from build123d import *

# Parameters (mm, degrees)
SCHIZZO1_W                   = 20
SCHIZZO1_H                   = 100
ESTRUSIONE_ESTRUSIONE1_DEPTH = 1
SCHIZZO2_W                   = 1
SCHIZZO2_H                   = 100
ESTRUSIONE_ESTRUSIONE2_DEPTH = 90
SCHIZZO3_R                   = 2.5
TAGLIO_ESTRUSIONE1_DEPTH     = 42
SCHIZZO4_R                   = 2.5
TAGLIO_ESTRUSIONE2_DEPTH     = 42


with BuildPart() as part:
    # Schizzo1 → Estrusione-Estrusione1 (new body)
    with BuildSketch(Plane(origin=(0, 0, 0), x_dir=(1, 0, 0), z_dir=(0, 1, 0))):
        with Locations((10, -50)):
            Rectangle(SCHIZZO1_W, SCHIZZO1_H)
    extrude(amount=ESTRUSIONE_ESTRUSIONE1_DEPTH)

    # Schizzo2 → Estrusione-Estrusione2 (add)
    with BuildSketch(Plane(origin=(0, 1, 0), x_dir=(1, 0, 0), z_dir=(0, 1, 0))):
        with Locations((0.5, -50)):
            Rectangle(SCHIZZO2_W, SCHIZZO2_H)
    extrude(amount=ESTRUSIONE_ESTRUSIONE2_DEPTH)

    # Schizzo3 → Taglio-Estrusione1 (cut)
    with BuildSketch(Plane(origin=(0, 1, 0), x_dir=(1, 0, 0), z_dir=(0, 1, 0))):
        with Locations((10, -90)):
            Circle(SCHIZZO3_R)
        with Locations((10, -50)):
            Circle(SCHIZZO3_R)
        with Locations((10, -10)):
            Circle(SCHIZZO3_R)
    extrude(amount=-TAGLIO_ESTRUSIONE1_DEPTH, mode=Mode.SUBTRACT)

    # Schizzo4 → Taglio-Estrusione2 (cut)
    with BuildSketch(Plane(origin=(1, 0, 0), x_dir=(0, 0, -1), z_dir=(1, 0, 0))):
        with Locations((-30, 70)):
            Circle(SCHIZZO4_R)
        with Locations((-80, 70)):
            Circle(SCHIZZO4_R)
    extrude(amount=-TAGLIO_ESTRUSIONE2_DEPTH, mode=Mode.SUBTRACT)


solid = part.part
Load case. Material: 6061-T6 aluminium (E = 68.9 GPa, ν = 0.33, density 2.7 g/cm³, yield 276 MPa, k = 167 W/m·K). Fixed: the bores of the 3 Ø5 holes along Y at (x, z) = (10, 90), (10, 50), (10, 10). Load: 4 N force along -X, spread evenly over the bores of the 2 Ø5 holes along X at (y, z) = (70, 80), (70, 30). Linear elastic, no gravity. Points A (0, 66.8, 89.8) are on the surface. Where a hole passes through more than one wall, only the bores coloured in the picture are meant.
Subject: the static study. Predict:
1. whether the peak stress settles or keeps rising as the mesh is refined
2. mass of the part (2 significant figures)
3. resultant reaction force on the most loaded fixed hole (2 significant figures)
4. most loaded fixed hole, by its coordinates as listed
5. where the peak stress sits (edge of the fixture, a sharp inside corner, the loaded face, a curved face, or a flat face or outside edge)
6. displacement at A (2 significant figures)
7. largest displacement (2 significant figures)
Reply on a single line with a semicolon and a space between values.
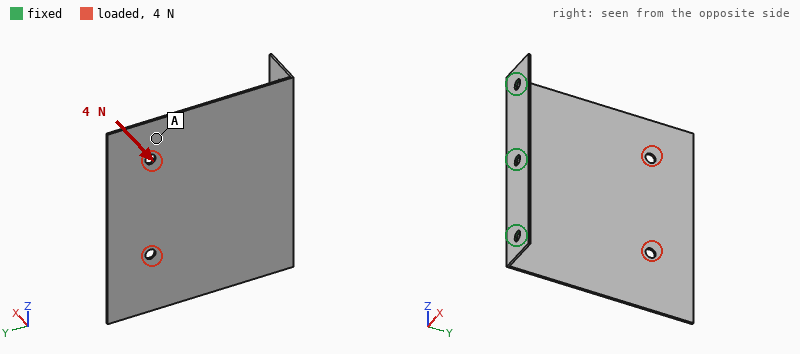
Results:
keeps rising; 29 g; 4.2 N; (10, 50); edge of the fixture; 0.95 mm; 1.4 mm
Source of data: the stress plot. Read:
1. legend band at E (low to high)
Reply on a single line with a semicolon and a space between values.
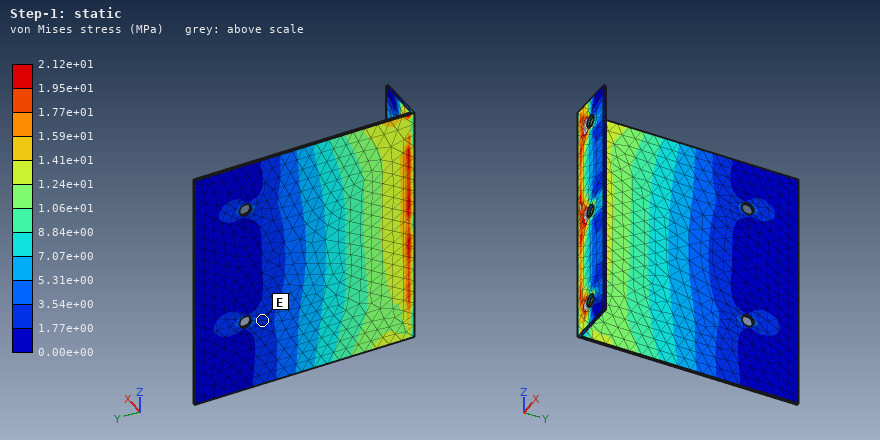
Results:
1.77e+00 to 3.54e+00 MPa
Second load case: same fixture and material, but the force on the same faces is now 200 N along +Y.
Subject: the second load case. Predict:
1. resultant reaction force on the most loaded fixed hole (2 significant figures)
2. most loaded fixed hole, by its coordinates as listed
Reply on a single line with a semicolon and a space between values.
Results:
78 N; (10, 90)
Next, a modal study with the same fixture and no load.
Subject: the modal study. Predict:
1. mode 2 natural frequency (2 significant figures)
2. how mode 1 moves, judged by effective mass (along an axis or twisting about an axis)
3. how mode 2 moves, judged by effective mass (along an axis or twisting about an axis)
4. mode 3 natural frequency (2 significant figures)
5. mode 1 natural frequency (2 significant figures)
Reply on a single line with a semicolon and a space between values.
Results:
220 Hz; along X; twisting about Y; 550 Hz; 88 Hz
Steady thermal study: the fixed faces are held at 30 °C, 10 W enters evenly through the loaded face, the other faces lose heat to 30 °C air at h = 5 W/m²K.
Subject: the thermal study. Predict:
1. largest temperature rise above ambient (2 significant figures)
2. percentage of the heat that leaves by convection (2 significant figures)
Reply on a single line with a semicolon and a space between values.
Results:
48 K; 25 %
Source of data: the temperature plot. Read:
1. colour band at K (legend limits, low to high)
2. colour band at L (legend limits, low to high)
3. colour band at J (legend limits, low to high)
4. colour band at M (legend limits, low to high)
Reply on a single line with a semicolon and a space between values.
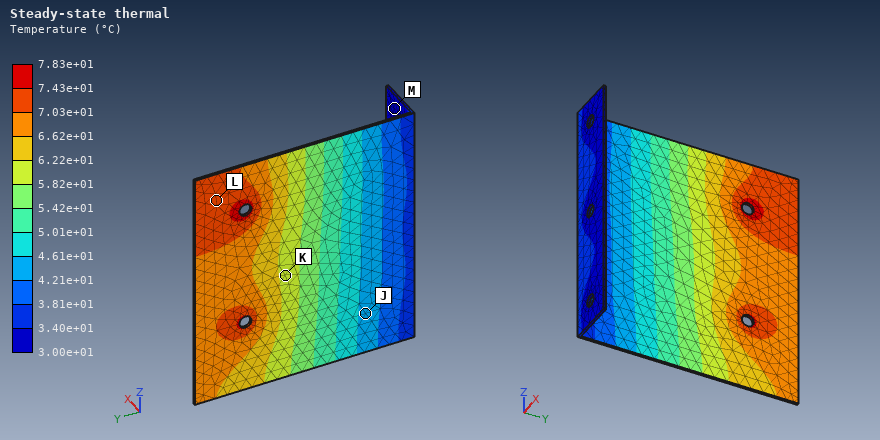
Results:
5.82e+01 to 6.22e+01 °C; 7.03e+01 to 7.43e+01 °C; 4.21e+01 to 4.61e+01 °C; 3.00e+01 to 3.40e+01 °C
